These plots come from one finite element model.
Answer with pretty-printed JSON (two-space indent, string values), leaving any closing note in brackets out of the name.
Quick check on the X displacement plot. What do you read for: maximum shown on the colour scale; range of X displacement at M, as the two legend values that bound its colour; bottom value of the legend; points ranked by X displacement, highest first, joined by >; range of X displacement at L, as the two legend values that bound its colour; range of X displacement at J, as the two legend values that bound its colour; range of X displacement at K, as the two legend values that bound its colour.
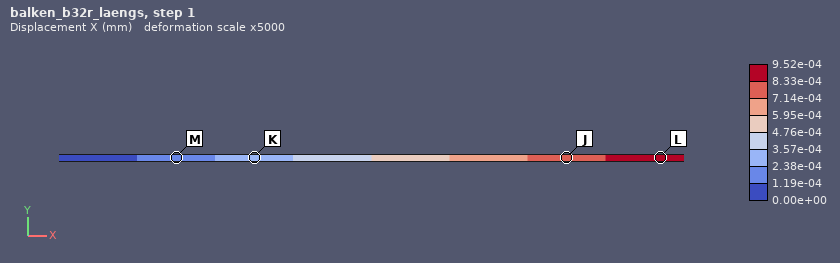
{
  "maximum shown on the colour scale": "9.52e-04 mm",
  "range of X displacement at M, as the two legend values that bound its colour": "1.19e-04 to 2.38e-04 mm",
  "bottom value of the legend": "0.00e+00 mm",
  "points ranked by X displacement, highest first, joined by >": "L > J > K > M",
  "range of X displacement at L, as the two legend values that bound its colour": "8.33e-04 to 9.52e-04 mm",
  "range of X displacement at J, as the two legend values that bound its colour": "7.14e-04 to 8.33e-04 mm",
  "range of X displacement at K, as the two legend values that bound its colour": "2.38e-04 to 3.57e-04 mm"
}
